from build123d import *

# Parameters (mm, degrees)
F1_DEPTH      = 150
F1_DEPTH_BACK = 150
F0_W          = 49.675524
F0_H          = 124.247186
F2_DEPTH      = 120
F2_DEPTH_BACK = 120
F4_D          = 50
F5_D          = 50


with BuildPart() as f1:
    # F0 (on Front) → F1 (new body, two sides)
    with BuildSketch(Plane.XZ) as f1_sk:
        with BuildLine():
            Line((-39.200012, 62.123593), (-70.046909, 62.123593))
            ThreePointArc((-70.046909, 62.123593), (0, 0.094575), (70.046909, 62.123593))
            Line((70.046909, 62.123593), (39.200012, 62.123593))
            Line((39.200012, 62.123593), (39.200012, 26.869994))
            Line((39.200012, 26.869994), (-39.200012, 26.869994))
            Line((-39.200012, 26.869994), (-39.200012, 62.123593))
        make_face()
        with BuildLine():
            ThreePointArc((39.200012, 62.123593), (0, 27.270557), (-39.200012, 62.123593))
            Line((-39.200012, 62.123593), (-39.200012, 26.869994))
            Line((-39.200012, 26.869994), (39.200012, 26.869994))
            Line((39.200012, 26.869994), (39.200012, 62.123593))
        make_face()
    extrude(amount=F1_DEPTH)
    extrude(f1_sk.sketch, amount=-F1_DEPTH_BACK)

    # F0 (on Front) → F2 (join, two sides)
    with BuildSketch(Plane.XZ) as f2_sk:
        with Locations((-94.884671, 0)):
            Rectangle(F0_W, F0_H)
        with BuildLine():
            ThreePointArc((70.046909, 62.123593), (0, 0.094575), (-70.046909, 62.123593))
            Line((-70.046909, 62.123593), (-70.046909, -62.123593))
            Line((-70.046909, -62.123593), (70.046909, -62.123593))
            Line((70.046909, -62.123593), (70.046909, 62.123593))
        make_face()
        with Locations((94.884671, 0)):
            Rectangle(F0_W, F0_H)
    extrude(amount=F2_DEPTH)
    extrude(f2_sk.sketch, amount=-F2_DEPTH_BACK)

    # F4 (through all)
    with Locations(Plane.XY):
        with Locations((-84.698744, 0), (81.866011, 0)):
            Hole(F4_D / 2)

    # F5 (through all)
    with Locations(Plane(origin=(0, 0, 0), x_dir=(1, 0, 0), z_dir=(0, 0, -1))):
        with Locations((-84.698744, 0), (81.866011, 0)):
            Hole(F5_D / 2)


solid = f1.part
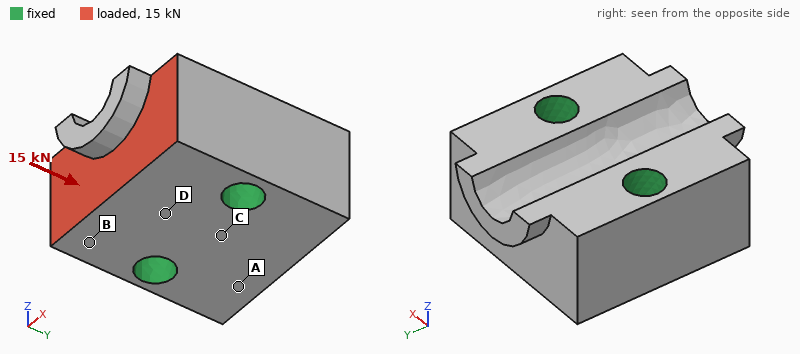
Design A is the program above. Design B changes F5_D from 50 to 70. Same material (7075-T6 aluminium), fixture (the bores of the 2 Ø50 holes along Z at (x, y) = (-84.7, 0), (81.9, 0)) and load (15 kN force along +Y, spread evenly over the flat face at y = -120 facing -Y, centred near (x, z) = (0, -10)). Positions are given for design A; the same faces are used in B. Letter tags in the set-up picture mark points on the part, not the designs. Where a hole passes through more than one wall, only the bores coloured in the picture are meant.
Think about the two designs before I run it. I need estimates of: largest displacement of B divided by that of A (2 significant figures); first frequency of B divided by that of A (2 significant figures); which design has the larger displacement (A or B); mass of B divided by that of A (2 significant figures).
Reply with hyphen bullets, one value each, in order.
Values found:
- 0.87
- 1.2
- A
- 0.93
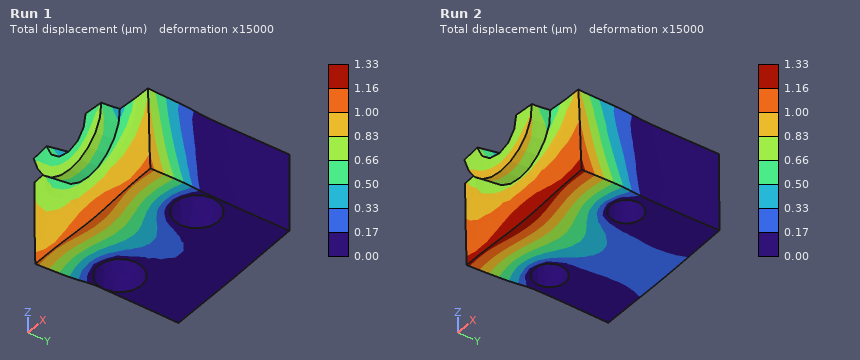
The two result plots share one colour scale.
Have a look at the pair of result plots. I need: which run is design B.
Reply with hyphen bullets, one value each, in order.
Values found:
- Run 1
